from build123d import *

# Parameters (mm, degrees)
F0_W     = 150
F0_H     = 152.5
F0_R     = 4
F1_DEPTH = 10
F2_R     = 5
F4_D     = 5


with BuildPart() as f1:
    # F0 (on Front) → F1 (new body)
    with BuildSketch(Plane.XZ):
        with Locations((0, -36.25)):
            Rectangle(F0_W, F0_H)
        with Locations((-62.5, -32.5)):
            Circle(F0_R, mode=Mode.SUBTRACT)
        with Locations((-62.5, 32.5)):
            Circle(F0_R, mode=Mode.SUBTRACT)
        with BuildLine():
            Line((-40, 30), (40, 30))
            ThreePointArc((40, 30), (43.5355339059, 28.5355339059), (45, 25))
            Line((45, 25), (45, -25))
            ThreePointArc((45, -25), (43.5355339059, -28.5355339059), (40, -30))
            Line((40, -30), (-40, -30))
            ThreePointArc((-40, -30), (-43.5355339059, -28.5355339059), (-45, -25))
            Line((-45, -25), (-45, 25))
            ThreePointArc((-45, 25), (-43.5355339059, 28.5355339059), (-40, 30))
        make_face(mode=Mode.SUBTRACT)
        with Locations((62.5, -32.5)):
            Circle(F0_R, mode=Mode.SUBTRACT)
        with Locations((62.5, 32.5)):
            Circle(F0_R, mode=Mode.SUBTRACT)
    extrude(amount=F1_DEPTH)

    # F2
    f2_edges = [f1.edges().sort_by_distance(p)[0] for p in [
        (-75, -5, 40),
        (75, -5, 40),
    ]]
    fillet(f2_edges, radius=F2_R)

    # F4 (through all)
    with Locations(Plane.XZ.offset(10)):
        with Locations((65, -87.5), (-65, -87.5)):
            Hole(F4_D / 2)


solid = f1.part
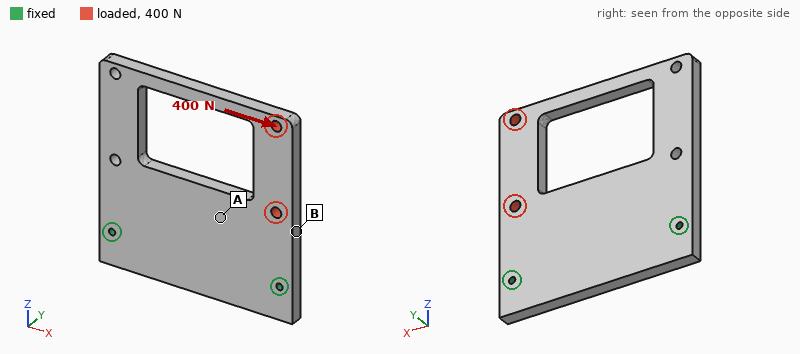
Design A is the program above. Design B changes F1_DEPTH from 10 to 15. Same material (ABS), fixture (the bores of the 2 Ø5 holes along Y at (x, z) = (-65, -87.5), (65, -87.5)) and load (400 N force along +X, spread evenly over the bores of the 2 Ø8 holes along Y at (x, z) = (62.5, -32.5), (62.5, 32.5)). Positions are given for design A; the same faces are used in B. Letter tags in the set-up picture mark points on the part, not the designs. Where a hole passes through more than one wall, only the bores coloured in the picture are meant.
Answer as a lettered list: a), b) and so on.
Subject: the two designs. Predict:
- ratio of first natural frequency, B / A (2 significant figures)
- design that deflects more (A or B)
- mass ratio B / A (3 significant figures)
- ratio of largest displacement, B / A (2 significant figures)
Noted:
a) 1.4
b) A
c) 1.50
d) 0.67
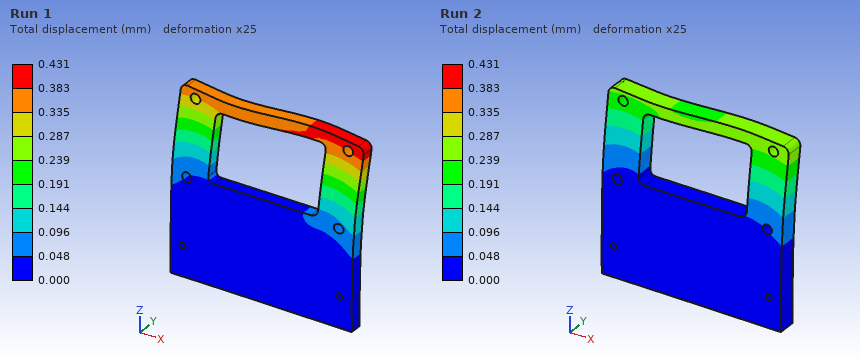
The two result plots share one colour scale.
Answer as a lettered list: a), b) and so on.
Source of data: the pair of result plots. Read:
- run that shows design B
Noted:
a) Run 2
